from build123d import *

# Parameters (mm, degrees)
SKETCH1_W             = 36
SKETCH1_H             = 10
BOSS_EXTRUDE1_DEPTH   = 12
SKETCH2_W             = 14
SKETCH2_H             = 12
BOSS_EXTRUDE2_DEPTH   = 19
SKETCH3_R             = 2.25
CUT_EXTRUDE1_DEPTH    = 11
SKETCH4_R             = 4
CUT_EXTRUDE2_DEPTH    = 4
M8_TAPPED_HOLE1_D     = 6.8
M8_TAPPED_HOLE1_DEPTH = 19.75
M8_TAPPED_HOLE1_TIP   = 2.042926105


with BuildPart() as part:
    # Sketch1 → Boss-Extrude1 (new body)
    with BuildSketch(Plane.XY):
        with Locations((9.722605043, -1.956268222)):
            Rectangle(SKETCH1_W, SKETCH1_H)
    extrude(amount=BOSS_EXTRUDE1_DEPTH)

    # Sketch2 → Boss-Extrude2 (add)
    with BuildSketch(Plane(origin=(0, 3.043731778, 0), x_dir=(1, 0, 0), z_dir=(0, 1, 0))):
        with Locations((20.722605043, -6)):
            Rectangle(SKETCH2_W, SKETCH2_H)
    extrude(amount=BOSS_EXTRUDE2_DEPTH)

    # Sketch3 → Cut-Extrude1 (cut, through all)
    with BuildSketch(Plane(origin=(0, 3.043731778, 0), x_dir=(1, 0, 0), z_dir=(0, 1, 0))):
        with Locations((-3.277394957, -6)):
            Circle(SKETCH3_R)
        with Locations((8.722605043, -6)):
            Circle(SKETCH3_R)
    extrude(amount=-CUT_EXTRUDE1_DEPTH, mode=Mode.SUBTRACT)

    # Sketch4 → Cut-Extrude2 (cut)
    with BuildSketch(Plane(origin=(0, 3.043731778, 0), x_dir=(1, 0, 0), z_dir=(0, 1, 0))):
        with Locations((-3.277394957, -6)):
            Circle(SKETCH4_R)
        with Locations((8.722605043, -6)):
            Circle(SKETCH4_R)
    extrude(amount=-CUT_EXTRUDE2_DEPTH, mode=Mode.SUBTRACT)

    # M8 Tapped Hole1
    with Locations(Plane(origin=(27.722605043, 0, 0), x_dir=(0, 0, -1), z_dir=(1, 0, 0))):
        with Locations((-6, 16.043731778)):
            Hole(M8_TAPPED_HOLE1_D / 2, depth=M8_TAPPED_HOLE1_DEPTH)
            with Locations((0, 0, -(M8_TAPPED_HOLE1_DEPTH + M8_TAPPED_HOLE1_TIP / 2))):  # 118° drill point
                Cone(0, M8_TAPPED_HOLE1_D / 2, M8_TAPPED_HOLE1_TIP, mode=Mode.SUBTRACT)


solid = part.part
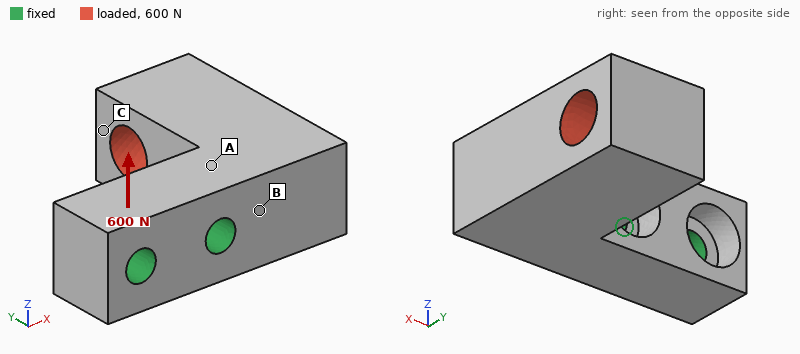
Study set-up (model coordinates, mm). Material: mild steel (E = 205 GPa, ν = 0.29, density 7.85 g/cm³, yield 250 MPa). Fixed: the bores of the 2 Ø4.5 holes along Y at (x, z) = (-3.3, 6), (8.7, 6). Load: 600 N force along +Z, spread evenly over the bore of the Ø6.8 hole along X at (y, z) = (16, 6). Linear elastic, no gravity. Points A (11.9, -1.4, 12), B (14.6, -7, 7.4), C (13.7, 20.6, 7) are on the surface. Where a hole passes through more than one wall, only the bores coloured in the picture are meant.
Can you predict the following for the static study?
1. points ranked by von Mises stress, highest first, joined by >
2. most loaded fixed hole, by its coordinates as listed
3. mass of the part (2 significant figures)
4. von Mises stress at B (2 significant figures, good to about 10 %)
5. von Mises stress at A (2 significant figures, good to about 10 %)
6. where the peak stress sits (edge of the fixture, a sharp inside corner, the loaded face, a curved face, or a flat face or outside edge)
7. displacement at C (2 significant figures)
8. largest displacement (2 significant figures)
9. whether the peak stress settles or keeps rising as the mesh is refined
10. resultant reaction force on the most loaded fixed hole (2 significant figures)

A > B > C
(8.7, 6)
50 g
43 MPa
78 MPa
edge of the fixture
26 µm
31 µm
keeps rising
820 N
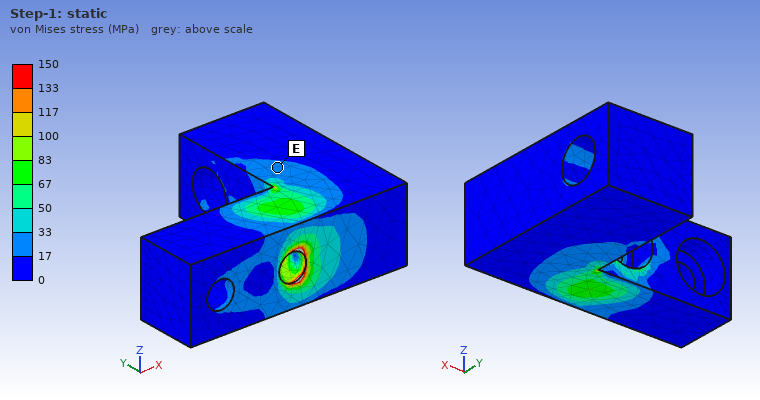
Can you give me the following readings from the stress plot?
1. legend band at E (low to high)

17 to 33 MPa
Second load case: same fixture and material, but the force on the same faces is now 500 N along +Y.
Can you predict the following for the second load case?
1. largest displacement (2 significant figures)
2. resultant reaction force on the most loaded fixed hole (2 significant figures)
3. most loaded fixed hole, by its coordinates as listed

10 µm
680 N
(8.7, 6)
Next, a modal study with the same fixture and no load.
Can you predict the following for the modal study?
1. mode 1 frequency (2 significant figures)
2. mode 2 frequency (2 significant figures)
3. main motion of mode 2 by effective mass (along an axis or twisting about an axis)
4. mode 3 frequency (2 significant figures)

6100 Hz
6500 Hz
along Z
15 kHz
